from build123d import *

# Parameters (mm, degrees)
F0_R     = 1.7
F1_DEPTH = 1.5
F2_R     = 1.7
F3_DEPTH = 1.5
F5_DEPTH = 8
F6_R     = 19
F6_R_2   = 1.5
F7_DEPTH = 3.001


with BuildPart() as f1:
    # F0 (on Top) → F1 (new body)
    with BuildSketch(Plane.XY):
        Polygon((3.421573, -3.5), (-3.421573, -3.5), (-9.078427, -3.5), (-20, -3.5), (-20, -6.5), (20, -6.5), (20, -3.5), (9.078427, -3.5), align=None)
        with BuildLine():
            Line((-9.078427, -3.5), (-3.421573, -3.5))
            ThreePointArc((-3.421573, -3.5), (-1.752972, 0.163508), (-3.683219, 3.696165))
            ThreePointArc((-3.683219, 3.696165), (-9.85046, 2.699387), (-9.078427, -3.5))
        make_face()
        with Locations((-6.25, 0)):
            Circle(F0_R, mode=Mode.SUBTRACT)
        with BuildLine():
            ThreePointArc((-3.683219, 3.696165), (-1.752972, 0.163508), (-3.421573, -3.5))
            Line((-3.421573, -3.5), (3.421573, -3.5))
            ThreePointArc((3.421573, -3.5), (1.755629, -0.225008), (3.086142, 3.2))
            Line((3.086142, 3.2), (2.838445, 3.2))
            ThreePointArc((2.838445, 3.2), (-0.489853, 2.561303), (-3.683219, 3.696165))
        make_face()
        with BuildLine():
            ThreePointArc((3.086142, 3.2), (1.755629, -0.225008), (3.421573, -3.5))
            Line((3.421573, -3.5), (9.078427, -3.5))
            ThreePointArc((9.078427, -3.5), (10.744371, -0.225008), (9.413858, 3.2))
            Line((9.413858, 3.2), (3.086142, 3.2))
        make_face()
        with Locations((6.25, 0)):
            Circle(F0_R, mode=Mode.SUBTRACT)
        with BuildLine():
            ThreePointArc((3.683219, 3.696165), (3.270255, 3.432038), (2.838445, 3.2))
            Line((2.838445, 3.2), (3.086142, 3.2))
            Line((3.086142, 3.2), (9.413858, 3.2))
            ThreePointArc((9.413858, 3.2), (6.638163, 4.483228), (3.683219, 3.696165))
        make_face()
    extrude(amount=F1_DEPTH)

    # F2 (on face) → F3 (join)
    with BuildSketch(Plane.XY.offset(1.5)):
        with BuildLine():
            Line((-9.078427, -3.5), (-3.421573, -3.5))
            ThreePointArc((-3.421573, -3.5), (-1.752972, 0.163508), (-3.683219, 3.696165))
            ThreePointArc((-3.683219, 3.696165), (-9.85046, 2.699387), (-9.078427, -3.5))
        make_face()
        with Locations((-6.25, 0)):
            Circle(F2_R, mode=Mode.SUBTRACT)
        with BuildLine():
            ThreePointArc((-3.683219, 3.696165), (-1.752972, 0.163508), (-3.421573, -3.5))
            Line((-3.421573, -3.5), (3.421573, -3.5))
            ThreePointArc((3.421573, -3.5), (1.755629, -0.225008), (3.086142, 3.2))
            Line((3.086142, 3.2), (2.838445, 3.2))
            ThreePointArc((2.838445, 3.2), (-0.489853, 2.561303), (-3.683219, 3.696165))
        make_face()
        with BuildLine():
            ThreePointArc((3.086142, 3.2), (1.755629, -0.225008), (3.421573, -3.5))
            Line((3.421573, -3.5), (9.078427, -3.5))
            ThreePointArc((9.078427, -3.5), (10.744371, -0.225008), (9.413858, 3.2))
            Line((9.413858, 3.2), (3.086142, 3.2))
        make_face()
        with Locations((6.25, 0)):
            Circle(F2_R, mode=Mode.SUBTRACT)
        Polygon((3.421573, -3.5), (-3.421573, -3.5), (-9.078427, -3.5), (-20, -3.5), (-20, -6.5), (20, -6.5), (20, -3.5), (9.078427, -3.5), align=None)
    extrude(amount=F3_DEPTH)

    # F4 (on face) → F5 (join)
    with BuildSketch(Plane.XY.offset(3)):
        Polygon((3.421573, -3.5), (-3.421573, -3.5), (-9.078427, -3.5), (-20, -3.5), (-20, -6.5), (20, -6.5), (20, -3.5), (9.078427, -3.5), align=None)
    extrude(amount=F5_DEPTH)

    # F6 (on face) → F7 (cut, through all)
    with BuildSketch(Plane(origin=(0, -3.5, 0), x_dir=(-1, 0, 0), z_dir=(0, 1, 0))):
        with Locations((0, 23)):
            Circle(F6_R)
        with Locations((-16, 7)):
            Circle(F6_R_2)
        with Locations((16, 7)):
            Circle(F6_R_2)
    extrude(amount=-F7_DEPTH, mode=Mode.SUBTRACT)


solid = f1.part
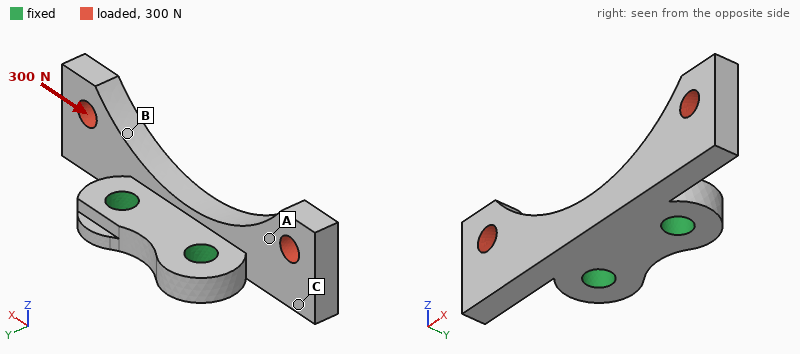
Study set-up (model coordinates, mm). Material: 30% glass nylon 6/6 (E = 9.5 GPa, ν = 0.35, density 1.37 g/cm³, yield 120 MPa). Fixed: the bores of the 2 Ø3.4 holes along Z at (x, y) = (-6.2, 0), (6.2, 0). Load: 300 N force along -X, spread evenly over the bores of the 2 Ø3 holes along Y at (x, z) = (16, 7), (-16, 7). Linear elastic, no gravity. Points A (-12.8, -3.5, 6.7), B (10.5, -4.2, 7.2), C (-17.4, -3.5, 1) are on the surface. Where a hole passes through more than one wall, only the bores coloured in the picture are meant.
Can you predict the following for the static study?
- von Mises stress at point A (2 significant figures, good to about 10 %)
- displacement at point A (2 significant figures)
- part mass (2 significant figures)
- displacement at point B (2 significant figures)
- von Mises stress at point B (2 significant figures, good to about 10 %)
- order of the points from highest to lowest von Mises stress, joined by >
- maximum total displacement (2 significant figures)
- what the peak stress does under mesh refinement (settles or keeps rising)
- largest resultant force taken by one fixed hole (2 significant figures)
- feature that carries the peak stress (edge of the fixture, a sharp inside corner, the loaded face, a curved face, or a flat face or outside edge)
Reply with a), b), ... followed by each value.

a) 11 MPa
b) 0.10 mm
c) 1.7 g
d) 0.089 mm
e) 26 MPa
f) B > A > C
g) 0.23 mm
h) keeps rising
i) 190 N
j) edge of the fixture
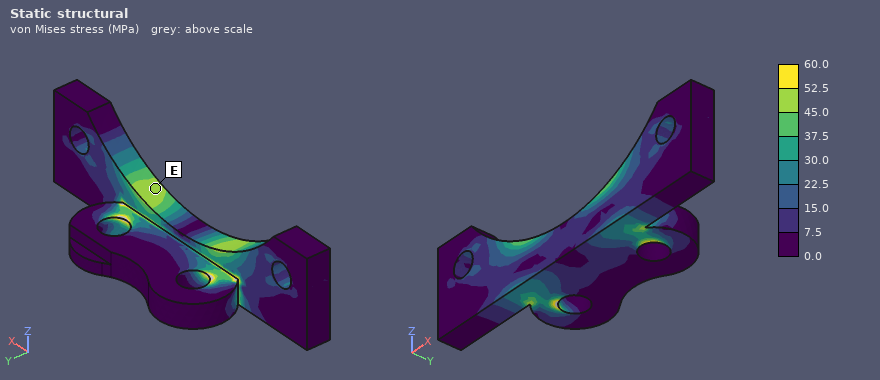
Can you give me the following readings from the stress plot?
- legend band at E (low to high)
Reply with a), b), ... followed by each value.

a) 45.0 to 52.5 MPa
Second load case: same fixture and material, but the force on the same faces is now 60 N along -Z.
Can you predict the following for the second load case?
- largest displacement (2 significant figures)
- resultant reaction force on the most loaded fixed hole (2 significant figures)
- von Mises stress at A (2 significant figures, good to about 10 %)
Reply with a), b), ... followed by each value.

a) 97 µm
b) 32 N
c) 2.4 MPa
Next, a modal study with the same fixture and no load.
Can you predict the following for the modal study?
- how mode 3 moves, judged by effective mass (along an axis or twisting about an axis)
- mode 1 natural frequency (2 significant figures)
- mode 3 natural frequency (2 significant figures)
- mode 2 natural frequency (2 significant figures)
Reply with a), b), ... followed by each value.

a) along Z
b) 4600 Hz
c) 6000 Hz
d) 4700 Hz
